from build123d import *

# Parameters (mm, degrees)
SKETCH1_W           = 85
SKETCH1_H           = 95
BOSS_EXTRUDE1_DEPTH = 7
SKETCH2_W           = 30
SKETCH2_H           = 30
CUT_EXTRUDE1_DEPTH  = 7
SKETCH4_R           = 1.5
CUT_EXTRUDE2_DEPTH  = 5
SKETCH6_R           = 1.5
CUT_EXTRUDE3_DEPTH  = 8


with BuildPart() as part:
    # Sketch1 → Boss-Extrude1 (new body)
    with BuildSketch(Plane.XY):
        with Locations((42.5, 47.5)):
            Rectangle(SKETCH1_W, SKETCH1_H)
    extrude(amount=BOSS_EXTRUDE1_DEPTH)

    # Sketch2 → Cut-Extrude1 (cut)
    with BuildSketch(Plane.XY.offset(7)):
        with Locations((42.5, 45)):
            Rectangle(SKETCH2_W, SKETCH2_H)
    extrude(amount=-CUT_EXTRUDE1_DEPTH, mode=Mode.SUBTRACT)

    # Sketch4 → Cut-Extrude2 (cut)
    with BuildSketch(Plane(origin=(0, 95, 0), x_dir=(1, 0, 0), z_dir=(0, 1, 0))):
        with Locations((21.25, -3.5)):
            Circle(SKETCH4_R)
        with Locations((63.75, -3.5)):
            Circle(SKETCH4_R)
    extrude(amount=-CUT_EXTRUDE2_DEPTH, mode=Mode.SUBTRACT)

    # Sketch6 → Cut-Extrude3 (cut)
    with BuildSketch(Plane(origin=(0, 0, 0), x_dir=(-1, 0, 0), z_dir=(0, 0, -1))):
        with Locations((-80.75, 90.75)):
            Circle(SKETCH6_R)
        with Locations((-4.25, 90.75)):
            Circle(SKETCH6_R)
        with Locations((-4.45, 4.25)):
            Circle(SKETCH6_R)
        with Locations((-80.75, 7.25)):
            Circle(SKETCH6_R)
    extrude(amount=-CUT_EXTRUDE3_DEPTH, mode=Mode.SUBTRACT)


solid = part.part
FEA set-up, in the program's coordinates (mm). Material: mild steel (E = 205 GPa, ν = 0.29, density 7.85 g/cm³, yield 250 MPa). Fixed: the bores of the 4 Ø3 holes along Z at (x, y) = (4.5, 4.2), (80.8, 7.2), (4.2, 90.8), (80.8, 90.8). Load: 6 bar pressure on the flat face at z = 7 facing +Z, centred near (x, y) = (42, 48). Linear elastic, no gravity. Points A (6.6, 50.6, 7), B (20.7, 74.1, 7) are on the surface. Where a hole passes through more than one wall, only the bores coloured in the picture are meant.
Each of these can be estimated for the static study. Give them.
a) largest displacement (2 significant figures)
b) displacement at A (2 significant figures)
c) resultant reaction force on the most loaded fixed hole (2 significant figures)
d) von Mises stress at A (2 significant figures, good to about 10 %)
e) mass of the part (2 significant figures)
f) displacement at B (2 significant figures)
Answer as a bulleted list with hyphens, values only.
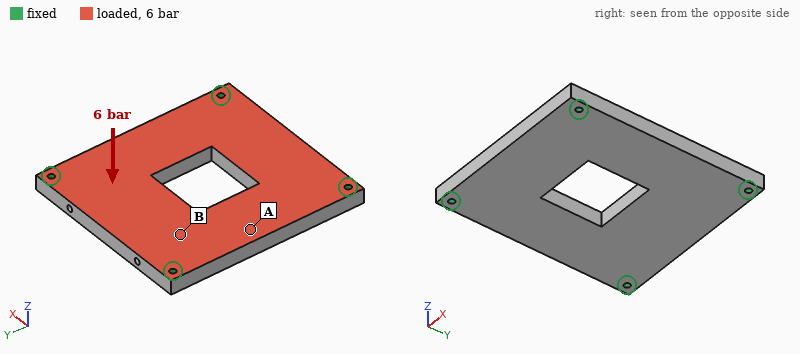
- 45 µm
- 30 µm
- 1.1 kN
- 34 MPa
- 390 g
- 25 µm
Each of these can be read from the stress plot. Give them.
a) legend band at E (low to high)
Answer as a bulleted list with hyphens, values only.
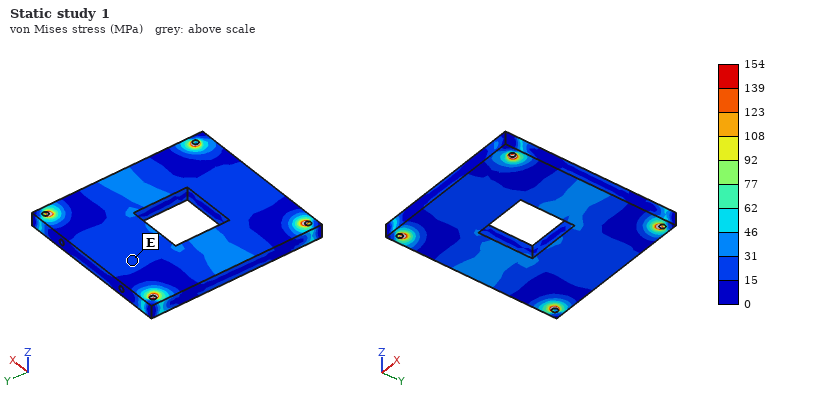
- 15 to 31 MPa
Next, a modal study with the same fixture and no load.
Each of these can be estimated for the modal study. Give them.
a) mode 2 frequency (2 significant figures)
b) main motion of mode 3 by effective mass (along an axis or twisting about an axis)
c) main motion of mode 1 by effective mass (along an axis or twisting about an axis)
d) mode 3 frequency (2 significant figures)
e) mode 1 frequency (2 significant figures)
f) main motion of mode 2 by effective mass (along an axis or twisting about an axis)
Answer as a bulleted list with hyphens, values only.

- 5100 Hz
- twisting about X
- along Z
- 5600 Hz
- 3100 Hz
- twisting about Y
